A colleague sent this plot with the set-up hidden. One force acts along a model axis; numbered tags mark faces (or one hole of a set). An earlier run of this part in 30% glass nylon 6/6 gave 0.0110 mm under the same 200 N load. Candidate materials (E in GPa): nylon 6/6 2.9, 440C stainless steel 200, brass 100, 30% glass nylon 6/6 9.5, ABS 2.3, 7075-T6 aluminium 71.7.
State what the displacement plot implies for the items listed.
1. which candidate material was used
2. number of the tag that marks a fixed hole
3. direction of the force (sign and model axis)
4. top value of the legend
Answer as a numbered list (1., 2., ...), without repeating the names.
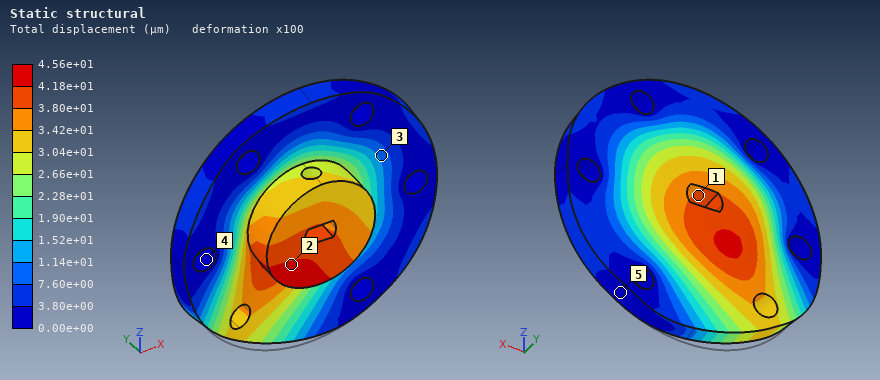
1. ABS
2. 4
3. +Y
4. 4.56e+01 µm
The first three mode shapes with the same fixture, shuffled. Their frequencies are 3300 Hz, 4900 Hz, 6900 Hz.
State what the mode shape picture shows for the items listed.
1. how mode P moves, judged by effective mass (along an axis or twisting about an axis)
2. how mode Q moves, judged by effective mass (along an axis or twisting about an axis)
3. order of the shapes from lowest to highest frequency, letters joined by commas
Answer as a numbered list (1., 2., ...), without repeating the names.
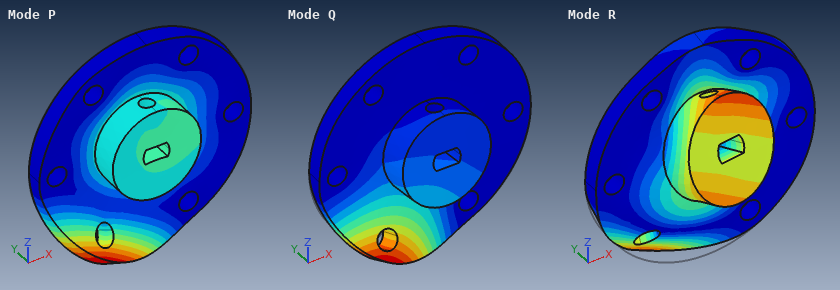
1. along Y
2. along Y
3. Q, P, R
